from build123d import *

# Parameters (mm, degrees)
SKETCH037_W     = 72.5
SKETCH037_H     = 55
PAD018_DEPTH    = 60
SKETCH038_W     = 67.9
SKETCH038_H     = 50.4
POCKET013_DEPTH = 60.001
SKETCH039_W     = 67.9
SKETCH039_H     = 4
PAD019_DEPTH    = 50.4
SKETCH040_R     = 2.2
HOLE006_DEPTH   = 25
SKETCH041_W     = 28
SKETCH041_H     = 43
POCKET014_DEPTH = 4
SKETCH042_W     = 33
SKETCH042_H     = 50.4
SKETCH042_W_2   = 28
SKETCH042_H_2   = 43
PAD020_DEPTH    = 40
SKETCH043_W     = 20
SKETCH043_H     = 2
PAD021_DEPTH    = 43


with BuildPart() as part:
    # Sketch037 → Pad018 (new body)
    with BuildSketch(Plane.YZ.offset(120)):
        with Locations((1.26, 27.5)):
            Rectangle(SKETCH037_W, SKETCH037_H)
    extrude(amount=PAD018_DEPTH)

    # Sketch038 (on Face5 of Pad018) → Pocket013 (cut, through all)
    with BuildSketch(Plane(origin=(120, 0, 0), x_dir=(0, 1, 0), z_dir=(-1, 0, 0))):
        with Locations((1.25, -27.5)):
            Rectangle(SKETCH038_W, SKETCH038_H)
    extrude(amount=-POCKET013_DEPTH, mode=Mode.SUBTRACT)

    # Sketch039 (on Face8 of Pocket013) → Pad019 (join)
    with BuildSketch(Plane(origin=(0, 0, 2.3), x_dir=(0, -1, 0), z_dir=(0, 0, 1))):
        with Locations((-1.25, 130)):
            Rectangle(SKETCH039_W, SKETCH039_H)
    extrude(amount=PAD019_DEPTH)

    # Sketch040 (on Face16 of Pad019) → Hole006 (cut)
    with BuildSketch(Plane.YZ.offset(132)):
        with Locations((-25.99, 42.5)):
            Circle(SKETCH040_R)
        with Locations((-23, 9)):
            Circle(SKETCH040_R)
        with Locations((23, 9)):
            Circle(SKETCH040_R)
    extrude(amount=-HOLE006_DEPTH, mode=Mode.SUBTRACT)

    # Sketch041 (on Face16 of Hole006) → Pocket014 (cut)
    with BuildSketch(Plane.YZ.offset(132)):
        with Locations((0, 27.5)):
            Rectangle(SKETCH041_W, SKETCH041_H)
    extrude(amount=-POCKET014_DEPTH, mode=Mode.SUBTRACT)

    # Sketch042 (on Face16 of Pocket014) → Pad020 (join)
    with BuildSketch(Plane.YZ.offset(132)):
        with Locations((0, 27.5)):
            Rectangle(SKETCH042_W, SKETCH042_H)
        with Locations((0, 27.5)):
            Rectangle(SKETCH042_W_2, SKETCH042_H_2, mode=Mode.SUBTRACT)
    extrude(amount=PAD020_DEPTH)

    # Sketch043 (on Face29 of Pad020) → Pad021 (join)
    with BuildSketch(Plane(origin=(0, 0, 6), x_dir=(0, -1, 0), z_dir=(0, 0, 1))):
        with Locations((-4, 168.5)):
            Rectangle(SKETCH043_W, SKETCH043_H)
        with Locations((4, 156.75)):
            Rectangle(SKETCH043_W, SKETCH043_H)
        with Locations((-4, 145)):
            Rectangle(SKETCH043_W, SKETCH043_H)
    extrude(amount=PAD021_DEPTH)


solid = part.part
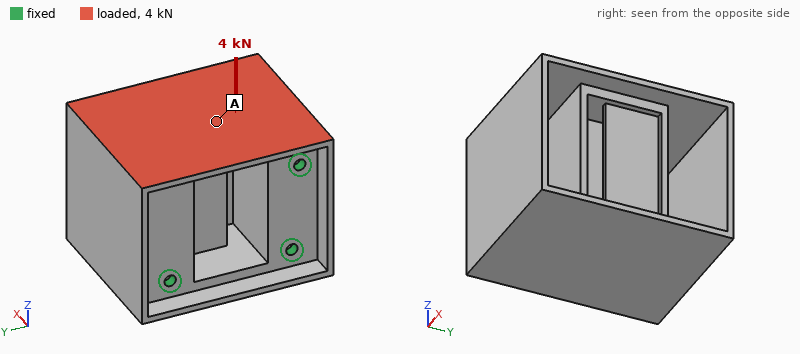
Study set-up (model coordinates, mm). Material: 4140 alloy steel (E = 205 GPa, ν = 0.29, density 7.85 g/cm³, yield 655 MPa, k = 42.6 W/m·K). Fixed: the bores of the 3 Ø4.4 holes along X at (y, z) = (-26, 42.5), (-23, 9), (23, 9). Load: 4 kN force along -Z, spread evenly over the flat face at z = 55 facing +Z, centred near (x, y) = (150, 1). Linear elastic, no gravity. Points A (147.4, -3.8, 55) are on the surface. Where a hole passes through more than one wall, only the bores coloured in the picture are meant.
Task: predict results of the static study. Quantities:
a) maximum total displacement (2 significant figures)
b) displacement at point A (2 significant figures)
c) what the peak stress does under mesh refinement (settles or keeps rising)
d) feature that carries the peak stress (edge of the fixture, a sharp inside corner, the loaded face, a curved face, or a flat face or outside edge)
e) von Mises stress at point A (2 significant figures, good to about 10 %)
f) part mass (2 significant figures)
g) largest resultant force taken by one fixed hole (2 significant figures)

55 µm
23 µm
keeps rising
edge of the fixture
7.9 MPa
520 g
2.5 kN
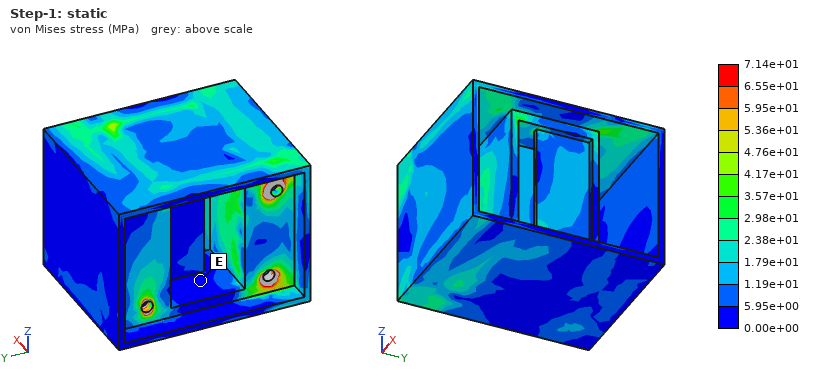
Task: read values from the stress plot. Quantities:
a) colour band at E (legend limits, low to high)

0.00e+00 to 5.95e+00 MPa
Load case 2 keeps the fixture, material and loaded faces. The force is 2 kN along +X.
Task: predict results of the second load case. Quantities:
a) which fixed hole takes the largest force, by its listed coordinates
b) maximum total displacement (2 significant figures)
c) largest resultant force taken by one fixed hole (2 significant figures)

(-26, 42.5)
60 µm
2.5 kN
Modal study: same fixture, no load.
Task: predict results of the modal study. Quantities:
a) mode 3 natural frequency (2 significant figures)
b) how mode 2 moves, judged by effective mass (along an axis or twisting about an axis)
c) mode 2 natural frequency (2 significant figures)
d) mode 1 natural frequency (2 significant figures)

4100 Hz
along Y
3800 Hz
2100 Hz
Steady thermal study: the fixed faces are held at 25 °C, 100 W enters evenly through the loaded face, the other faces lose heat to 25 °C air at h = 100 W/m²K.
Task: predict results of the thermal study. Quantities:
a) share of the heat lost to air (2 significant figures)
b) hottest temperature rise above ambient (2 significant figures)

81 %
67 K
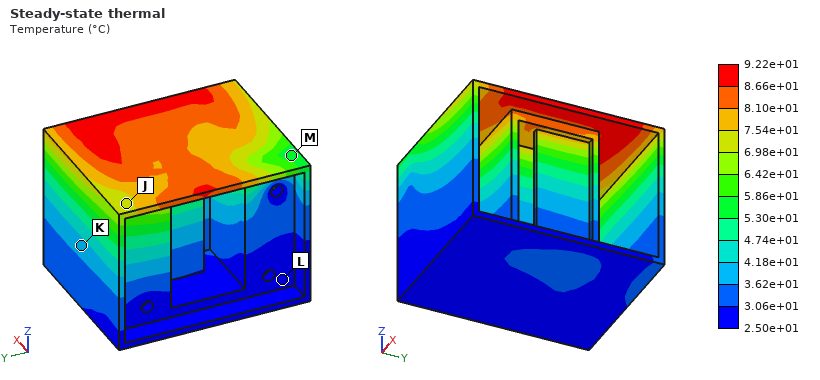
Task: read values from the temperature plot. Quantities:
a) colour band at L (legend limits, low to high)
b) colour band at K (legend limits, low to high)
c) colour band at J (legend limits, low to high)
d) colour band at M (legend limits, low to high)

2.50e+01 to 3.06e+01 °C
3.62e+01 to 4.18e+01 °C
6.98e+01 to 7.54e+01 °C
5.30e+01 to 5.86e+01 °C
